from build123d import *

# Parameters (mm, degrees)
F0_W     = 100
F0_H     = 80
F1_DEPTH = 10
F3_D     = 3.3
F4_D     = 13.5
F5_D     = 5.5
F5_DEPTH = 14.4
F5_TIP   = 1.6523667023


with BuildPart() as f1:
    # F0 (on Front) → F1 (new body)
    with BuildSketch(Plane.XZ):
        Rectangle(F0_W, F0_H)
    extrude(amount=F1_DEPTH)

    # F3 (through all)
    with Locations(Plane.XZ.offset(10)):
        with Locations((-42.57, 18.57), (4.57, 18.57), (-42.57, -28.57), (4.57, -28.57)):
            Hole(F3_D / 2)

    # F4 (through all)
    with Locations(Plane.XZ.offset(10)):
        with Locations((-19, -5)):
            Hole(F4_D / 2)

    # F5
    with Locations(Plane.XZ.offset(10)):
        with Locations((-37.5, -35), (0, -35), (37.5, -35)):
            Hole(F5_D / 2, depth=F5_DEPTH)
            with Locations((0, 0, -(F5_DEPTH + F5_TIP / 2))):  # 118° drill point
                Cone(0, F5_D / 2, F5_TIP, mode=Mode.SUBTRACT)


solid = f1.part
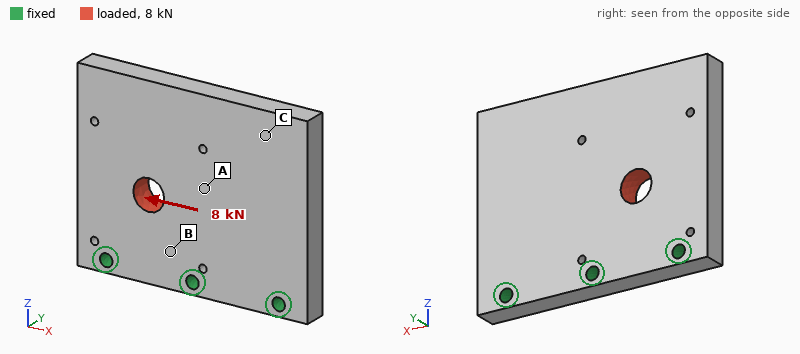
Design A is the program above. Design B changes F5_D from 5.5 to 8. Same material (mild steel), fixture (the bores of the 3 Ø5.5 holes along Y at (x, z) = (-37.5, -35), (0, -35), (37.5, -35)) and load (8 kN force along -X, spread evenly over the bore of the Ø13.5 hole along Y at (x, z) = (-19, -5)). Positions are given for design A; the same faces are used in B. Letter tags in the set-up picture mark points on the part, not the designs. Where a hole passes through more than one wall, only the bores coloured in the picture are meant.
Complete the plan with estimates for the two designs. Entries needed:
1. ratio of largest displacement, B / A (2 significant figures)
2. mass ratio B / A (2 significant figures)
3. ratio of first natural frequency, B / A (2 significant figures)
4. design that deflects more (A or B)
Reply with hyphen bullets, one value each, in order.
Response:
- 0.88
- 0.99
- 1.1
- A
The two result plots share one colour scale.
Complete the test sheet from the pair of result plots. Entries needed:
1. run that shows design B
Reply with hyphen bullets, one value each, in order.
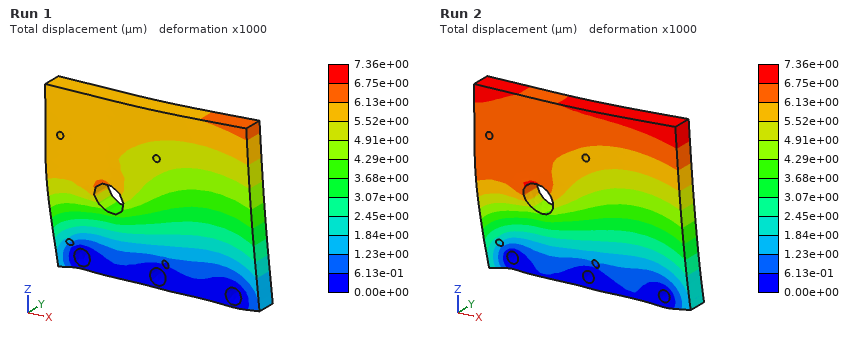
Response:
- Run 1
